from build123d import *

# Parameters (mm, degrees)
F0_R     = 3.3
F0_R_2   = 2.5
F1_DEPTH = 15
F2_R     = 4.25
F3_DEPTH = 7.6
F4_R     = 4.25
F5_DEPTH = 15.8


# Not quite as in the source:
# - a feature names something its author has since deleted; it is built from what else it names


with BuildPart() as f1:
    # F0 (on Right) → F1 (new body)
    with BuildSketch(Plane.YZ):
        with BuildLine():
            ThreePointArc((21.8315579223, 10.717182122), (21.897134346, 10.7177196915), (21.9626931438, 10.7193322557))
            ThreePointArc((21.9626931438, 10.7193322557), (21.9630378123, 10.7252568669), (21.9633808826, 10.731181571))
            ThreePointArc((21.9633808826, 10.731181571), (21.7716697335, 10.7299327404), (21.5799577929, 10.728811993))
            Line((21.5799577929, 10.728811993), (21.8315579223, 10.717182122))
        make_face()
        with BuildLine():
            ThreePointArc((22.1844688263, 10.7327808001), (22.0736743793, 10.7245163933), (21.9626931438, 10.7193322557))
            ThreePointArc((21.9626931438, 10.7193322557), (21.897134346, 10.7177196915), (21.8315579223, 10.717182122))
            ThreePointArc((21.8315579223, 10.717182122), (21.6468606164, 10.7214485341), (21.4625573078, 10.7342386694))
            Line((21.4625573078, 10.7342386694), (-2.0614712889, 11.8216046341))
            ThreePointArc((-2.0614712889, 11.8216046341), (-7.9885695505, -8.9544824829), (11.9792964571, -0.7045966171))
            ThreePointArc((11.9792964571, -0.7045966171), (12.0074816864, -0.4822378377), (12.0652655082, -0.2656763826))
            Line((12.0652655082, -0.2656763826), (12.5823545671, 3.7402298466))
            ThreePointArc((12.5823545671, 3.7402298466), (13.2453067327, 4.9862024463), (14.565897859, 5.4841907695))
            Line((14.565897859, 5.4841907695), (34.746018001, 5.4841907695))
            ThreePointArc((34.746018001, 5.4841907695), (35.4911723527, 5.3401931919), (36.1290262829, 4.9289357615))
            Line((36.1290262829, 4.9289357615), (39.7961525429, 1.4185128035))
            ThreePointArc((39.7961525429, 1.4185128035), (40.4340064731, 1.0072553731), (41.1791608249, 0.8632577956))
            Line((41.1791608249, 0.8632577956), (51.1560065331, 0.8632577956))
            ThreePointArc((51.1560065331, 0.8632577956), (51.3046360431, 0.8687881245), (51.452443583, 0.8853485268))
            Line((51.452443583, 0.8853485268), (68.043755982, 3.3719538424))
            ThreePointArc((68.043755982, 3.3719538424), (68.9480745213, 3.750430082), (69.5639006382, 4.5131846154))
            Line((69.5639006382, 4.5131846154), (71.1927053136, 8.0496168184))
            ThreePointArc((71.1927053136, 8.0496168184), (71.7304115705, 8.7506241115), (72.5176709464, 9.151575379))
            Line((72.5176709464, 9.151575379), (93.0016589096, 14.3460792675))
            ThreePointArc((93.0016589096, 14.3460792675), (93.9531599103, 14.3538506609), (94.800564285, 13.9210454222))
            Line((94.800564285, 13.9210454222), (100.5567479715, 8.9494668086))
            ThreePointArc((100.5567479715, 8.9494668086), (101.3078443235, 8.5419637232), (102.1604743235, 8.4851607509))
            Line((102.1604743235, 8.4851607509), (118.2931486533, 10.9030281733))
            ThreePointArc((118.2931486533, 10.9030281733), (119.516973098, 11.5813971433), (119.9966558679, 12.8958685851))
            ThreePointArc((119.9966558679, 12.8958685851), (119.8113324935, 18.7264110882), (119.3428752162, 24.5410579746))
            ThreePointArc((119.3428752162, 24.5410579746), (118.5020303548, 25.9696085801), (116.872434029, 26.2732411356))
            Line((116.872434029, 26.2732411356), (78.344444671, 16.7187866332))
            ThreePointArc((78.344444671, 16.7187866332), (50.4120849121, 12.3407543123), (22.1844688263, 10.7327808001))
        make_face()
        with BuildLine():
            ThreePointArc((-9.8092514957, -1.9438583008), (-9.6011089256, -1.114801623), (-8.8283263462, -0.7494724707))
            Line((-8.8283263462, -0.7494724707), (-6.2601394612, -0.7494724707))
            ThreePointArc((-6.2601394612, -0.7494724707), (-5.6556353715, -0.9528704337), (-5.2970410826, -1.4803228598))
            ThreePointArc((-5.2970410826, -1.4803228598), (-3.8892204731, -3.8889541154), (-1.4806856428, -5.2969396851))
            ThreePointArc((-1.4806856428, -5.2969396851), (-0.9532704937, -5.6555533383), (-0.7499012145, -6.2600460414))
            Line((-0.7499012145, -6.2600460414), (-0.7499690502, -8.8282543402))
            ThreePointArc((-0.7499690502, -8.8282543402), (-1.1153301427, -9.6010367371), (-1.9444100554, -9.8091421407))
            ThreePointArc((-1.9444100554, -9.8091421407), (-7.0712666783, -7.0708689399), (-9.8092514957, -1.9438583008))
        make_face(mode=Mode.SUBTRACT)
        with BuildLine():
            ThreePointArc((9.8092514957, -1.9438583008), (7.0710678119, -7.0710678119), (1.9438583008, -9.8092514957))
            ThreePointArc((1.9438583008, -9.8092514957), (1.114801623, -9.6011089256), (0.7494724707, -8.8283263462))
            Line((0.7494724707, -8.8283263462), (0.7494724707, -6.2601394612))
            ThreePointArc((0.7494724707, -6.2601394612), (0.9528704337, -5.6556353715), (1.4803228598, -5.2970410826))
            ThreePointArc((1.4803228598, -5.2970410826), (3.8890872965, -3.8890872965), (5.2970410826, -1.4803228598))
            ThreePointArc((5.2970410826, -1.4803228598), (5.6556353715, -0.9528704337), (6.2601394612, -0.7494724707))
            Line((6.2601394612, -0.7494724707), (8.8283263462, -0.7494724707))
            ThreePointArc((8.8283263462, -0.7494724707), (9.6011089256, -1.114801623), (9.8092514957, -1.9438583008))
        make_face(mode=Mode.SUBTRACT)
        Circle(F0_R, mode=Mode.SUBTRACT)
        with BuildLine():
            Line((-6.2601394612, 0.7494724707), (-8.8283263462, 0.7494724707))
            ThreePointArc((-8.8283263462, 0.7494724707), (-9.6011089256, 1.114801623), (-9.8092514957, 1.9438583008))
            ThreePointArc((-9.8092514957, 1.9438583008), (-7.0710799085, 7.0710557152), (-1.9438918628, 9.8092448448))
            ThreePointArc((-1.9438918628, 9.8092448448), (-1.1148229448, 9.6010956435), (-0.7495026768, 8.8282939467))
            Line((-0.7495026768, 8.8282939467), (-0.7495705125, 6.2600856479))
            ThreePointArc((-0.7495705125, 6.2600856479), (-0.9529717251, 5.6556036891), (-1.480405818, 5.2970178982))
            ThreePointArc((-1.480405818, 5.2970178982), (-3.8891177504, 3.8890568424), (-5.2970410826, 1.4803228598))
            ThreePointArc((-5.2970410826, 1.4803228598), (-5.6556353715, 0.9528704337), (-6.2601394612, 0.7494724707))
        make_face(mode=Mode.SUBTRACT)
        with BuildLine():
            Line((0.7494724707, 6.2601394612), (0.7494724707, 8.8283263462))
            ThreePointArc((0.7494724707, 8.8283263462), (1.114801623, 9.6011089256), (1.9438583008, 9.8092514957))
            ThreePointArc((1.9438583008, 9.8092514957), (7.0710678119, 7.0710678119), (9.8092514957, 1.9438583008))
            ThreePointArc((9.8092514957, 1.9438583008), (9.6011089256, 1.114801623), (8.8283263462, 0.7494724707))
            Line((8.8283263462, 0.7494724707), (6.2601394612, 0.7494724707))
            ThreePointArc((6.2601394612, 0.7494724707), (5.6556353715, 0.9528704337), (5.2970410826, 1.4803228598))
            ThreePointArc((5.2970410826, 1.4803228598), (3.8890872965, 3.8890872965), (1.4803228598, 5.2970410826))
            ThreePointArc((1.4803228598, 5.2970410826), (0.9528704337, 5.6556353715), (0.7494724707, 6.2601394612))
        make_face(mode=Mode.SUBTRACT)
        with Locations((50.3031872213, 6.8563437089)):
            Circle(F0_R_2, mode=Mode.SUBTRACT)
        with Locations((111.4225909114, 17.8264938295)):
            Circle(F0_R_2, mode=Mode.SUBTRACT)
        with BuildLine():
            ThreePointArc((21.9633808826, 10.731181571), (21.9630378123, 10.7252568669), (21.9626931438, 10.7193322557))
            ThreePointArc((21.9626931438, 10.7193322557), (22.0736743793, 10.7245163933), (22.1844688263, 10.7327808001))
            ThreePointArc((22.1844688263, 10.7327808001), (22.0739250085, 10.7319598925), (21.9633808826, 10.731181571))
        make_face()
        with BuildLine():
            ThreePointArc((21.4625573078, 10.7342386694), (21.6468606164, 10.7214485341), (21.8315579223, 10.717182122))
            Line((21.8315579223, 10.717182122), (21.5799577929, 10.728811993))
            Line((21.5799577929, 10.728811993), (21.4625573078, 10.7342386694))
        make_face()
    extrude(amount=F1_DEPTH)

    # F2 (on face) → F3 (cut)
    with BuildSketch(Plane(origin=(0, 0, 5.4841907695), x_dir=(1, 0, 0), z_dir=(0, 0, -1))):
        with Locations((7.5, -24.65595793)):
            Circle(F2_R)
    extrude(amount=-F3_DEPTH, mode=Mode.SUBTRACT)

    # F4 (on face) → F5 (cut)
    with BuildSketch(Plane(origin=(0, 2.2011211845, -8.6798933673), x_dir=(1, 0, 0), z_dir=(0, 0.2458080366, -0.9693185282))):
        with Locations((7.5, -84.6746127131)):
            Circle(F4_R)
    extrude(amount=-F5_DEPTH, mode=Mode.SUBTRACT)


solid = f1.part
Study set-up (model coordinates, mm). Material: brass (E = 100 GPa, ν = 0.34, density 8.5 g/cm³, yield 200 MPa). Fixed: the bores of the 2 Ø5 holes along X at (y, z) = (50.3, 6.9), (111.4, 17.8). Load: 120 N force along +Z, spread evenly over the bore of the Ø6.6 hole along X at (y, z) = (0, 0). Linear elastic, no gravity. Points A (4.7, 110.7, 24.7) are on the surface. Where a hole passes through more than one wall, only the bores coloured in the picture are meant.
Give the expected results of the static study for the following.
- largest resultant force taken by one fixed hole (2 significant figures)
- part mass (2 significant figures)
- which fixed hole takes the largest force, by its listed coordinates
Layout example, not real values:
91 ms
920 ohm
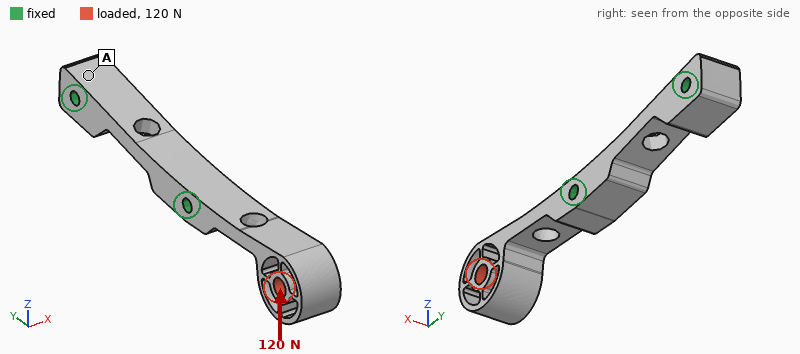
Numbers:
130 N
150 g
(50.3, 6.9)
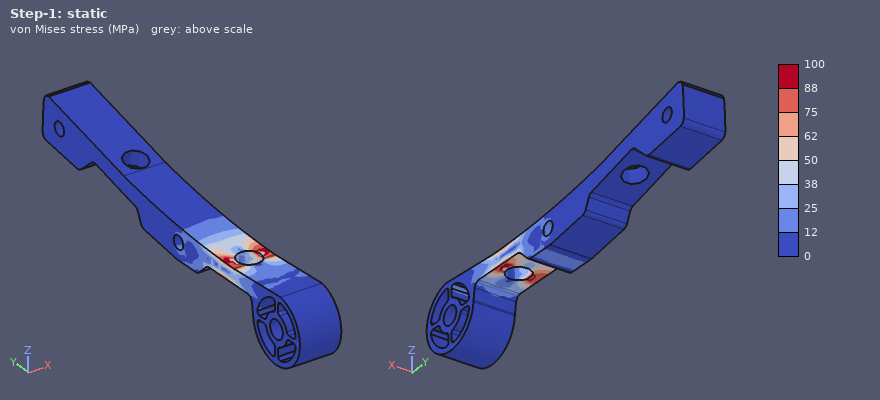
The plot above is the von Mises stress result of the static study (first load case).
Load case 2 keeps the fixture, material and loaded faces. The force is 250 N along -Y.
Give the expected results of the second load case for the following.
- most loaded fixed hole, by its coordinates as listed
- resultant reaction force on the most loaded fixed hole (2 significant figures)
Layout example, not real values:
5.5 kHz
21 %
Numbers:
(50.3, 6.9)
250 N
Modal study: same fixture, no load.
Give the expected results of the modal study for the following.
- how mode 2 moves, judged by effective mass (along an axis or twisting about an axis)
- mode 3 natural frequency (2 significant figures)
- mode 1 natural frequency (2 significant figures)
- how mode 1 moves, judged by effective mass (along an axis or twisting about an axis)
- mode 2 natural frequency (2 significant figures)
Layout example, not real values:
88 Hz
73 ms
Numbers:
along X
3200 Hz
680 Hz
along Z
1400 Hz
